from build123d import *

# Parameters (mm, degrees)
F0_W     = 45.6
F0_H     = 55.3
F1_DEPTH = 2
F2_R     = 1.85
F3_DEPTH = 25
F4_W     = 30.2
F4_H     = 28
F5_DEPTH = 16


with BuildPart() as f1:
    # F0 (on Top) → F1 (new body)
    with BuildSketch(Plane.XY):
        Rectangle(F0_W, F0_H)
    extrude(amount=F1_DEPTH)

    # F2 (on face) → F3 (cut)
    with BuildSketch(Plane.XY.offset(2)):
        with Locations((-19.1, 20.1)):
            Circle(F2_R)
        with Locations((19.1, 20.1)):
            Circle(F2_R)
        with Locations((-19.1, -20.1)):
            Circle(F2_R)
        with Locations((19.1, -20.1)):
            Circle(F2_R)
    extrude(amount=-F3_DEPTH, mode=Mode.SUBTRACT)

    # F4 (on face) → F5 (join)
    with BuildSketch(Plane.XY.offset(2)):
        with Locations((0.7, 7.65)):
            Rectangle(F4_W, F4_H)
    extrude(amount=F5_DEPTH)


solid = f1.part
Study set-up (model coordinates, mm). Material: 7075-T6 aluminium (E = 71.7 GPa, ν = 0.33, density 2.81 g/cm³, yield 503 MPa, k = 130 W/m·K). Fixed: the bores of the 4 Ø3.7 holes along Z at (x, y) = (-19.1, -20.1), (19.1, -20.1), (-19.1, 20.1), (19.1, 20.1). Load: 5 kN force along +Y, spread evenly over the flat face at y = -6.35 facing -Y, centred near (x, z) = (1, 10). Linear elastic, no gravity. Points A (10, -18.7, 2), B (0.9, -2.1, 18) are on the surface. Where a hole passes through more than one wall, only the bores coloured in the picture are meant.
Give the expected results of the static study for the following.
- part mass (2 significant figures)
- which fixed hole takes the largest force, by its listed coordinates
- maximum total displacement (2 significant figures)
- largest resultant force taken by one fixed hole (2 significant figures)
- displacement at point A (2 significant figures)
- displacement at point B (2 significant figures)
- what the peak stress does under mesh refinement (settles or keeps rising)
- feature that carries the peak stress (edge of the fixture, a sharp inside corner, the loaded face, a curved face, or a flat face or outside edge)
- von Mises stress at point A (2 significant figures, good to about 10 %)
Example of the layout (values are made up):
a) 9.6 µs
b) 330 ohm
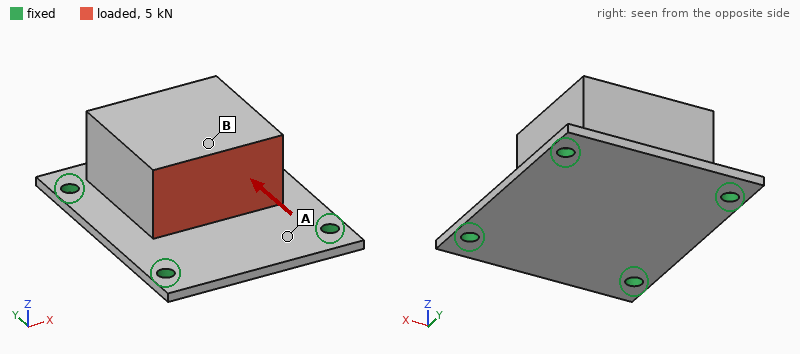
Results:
a) 52 g
b) (19.1, 20.1)
c) 0.25 mm
d) 1.7 kN
e) 0.068 mm
f) 0.22 mm
g) keeps rising
h) edge of the fixture
i) 64 MPa
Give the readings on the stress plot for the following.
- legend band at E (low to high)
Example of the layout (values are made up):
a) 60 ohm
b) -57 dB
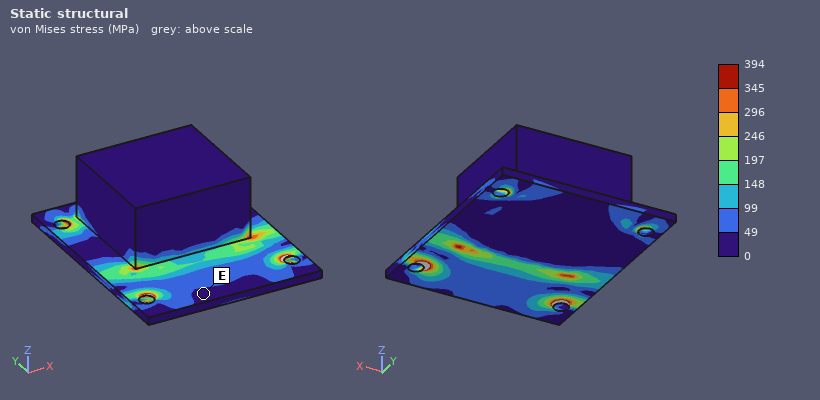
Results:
a) 0 to 49 MPa
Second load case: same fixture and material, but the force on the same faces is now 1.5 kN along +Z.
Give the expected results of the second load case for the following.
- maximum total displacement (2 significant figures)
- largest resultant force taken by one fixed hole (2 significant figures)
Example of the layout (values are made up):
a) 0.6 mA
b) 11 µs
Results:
a) 0.21 mm
b) 550 N
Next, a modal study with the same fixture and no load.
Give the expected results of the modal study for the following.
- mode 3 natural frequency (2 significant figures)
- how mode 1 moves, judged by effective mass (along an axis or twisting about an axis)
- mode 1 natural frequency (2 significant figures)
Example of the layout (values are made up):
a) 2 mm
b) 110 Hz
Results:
a) 9100 Hz
b) along Z
c) 3200 Hz
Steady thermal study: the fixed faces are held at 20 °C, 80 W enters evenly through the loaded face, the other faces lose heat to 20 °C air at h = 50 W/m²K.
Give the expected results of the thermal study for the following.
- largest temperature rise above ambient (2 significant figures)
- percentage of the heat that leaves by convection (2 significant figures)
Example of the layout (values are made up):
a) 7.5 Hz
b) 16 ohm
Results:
a) 60 K
b) 14 %
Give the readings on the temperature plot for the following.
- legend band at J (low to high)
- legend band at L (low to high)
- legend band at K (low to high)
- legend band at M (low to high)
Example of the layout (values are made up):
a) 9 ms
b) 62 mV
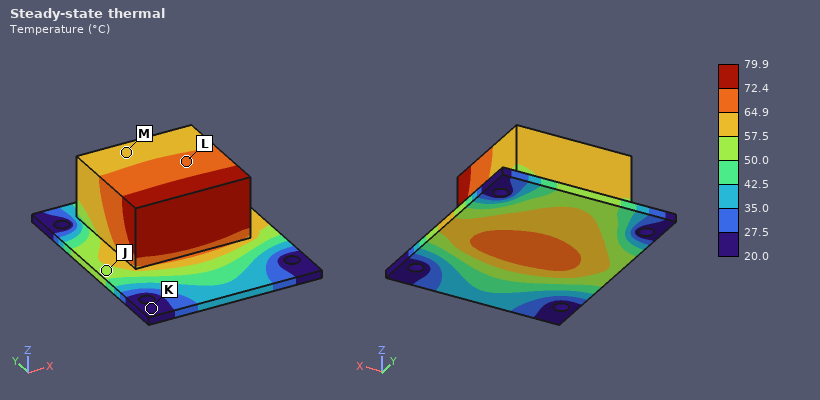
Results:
a) 50.0 to 57.5 °C
b) 64.9 to 72.4 °C
c) 20.0 to 27.5 °C
d) 57.5 to 64.9 °C
